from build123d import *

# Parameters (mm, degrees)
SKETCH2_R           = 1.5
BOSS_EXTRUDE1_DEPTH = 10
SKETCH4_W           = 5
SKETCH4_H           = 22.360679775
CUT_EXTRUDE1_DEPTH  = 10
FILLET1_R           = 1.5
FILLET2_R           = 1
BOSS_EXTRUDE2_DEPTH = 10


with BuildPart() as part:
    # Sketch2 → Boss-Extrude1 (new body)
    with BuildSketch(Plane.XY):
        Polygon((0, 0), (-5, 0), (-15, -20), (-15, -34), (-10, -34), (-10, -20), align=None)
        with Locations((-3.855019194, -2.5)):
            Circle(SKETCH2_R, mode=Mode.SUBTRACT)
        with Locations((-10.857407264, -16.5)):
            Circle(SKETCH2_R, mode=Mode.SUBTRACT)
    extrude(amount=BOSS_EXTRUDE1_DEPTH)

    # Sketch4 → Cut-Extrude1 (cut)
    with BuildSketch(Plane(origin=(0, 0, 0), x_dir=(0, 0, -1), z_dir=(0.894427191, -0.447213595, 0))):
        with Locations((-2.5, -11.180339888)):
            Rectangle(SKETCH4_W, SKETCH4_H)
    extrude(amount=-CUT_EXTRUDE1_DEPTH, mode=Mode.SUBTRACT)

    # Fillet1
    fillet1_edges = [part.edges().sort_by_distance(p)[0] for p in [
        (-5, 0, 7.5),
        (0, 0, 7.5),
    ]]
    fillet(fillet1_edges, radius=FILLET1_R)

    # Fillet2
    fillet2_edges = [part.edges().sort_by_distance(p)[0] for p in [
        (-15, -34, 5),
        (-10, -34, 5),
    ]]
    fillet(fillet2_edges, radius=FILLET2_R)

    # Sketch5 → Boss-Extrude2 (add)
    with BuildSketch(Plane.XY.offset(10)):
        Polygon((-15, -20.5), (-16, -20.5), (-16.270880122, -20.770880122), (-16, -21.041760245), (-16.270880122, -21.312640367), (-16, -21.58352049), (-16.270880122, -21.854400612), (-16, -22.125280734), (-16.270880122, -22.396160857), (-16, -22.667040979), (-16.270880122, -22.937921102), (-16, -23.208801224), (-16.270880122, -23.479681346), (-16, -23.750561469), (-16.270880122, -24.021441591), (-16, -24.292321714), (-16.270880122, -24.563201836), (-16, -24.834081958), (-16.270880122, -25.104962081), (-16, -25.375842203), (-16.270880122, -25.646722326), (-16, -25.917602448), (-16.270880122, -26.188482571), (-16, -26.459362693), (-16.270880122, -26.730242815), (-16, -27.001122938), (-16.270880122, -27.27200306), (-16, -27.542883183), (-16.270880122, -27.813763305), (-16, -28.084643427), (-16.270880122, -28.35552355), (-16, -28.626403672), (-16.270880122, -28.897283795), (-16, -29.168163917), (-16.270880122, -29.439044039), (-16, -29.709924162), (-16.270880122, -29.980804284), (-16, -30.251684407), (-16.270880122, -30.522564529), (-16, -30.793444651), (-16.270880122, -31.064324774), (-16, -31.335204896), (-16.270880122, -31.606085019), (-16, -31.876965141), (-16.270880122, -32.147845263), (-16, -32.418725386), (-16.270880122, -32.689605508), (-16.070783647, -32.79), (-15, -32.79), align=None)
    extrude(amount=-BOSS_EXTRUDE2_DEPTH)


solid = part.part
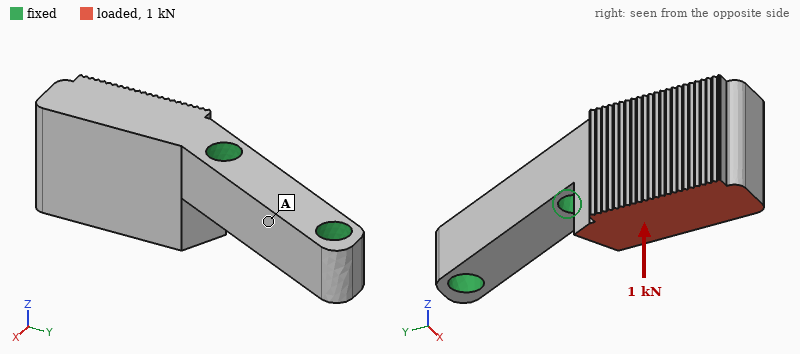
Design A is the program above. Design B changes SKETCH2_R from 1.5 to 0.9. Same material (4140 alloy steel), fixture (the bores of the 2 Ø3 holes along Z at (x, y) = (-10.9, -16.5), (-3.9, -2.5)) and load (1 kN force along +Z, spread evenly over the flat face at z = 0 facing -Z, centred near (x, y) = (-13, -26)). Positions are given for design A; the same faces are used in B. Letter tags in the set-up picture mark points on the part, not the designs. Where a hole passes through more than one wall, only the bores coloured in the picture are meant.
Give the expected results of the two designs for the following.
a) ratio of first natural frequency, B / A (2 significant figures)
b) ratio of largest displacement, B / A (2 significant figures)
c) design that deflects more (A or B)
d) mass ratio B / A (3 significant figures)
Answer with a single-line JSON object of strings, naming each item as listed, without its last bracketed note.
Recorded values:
{"ratio of first natural frequency, B / A": "0.84", "ratio of largest displacement, B / A": "1.3", "design that deflects more": "B", "mass ratio B / A": "1.04"}
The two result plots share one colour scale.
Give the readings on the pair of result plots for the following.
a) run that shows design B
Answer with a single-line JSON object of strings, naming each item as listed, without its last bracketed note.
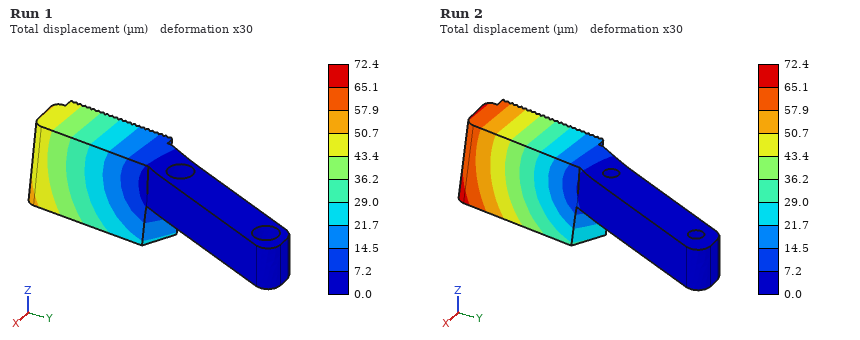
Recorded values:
{"run that shows design B": "Run 2"}
